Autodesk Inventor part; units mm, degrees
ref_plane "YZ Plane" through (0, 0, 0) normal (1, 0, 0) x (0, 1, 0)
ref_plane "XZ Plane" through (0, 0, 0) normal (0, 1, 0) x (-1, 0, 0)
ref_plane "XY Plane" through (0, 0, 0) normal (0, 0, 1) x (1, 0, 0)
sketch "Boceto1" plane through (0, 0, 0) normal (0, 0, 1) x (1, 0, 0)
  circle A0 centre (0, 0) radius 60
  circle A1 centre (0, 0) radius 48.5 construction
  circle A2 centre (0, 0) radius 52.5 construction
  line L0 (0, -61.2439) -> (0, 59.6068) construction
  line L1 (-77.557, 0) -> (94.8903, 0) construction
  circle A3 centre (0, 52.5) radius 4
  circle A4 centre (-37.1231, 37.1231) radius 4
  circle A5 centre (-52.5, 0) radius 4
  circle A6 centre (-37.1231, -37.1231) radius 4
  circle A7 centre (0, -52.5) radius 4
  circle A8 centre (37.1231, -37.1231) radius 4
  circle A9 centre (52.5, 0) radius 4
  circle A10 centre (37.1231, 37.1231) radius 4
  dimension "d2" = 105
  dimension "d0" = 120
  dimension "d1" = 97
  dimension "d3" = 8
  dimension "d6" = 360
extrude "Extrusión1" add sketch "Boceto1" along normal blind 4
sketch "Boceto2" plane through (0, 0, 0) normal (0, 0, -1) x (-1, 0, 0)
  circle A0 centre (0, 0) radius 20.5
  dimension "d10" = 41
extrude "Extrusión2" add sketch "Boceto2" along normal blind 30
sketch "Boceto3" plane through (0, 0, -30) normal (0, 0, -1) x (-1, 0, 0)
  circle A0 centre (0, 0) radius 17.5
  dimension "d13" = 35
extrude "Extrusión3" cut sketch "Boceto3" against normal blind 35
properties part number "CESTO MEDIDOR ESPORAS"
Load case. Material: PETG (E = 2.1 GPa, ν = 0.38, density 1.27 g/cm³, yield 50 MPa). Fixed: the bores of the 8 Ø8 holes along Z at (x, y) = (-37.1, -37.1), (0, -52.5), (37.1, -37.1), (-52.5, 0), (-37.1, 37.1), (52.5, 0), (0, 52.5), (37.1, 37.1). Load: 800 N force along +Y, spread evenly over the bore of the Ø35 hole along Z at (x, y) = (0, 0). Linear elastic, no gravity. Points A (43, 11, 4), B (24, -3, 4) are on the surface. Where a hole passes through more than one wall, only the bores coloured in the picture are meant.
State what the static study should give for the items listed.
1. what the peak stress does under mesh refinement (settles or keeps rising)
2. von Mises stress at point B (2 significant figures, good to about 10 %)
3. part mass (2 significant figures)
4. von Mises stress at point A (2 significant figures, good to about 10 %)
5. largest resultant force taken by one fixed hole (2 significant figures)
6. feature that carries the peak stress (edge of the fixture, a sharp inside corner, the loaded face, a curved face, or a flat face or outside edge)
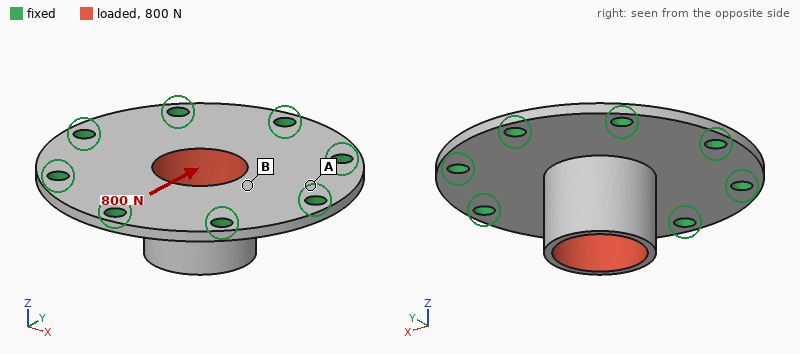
keeps rising
6.0 MPa
64 g
2.3 MPa
190 N
edge of the fixture
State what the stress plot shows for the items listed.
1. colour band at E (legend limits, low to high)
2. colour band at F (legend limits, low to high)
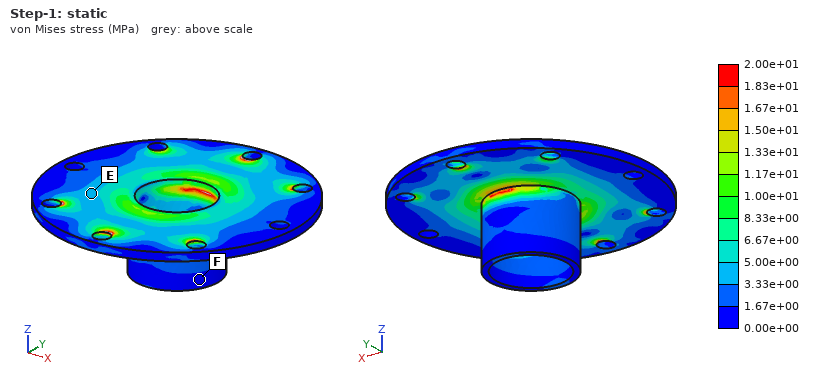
3.33e+00 to 5.00e+00 MPa
0.00e+00 to 1.67e+00 MPa
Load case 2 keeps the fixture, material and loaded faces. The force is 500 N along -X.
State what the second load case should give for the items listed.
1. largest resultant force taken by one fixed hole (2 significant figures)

120 N
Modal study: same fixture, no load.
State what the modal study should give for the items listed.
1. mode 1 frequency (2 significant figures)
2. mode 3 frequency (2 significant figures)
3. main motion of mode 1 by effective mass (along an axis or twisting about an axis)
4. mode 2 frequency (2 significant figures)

860 Hz
1000 Hz
along Z
1000 Hz
